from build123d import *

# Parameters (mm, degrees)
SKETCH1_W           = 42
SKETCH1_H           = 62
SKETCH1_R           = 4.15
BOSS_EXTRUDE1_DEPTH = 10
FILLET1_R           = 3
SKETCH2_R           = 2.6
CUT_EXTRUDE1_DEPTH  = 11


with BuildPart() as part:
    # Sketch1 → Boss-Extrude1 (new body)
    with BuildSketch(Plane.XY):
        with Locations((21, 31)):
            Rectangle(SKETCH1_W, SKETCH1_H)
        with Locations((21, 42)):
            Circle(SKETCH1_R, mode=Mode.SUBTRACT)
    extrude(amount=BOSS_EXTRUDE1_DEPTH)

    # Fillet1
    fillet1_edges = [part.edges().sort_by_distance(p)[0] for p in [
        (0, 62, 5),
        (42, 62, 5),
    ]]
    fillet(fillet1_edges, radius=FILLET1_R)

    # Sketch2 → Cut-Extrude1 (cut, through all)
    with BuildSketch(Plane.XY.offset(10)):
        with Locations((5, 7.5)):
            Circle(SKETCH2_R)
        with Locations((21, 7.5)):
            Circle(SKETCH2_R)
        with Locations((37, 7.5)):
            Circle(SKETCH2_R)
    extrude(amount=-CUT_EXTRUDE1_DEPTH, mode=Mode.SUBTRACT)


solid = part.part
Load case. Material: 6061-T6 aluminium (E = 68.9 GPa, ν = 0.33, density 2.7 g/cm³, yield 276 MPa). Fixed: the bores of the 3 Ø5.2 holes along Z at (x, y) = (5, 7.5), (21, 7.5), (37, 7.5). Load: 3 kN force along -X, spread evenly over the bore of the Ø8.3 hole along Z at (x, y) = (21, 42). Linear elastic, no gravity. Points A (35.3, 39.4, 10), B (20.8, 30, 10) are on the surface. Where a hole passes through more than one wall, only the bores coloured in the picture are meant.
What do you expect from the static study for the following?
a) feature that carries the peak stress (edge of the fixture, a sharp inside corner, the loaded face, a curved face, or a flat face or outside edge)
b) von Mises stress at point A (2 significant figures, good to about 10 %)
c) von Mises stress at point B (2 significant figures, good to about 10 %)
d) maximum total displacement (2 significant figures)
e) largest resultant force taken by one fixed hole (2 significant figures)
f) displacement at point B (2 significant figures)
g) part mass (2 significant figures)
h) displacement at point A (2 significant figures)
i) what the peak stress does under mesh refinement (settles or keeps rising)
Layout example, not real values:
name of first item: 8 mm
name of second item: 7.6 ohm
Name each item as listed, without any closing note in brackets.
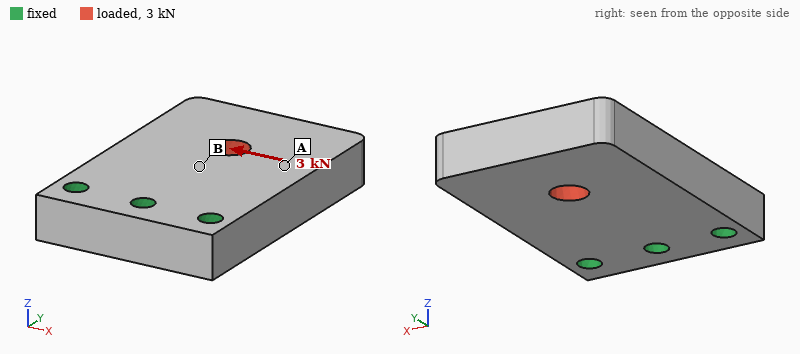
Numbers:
feature that carries the peak stress: edge of the fixture
von Mises stress at point A: 9.8 MPa
von Mises stress at point B: 20 MPa
maximum total displacement: 30 µm
largest resultant force taken by one fixed hole: 3.1 kN
displacement at point B: 11 µm
part mass: 67 g
displacement at point A: 18 µm
what the peak stress does under mesh refinement: keeps rising
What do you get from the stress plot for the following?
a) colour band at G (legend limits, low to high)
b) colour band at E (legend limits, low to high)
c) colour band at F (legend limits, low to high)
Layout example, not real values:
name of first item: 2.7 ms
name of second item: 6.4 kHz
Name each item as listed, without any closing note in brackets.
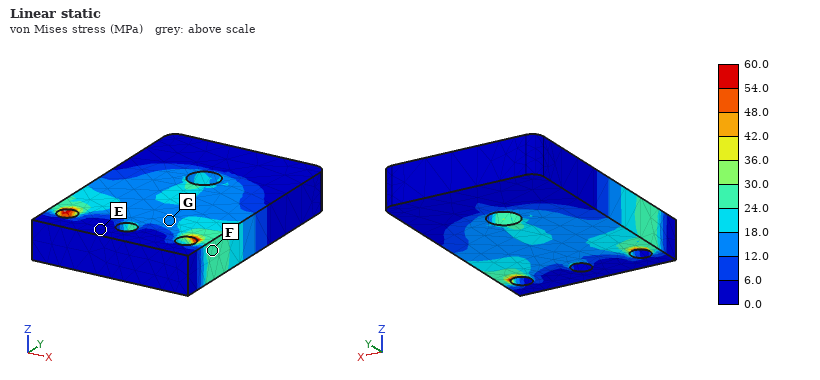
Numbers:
colour band at G: 12.0 to 18.0 MPa
colour band at E: 0.0 to 6.0 MPa
colour band at F: 24.0 to 30.0 MPa
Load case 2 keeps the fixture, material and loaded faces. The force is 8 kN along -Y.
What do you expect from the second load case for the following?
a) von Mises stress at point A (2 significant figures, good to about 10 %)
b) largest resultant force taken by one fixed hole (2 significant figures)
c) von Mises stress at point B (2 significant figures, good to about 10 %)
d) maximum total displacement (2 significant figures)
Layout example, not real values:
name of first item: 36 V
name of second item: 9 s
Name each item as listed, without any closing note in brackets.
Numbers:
von Mises stress at point A: 11 MPa
largest resultant force taken by one fixed hole: 2.8 kN
von Mises stress at point B: 28 MPa
maximum total displacement: 15 µm
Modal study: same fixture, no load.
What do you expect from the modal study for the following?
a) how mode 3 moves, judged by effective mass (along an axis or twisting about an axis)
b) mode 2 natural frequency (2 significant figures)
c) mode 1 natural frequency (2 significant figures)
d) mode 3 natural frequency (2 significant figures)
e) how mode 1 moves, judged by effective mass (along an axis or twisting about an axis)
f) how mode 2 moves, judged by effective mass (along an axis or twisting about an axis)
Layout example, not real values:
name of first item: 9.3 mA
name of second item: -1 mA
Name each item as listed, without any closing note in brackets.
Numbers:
how mode 3 moves, judged by effective mass: along X
mode 2 natural frequency: 7200 Hz
mode 1 natural frequency: 2800 Hz
mode 3 natural frequency: 8600 Hz
how mode 1 moves, judged by effective mass: along Z
how mode 2 moves, judged by effective mass: twisting about Y
